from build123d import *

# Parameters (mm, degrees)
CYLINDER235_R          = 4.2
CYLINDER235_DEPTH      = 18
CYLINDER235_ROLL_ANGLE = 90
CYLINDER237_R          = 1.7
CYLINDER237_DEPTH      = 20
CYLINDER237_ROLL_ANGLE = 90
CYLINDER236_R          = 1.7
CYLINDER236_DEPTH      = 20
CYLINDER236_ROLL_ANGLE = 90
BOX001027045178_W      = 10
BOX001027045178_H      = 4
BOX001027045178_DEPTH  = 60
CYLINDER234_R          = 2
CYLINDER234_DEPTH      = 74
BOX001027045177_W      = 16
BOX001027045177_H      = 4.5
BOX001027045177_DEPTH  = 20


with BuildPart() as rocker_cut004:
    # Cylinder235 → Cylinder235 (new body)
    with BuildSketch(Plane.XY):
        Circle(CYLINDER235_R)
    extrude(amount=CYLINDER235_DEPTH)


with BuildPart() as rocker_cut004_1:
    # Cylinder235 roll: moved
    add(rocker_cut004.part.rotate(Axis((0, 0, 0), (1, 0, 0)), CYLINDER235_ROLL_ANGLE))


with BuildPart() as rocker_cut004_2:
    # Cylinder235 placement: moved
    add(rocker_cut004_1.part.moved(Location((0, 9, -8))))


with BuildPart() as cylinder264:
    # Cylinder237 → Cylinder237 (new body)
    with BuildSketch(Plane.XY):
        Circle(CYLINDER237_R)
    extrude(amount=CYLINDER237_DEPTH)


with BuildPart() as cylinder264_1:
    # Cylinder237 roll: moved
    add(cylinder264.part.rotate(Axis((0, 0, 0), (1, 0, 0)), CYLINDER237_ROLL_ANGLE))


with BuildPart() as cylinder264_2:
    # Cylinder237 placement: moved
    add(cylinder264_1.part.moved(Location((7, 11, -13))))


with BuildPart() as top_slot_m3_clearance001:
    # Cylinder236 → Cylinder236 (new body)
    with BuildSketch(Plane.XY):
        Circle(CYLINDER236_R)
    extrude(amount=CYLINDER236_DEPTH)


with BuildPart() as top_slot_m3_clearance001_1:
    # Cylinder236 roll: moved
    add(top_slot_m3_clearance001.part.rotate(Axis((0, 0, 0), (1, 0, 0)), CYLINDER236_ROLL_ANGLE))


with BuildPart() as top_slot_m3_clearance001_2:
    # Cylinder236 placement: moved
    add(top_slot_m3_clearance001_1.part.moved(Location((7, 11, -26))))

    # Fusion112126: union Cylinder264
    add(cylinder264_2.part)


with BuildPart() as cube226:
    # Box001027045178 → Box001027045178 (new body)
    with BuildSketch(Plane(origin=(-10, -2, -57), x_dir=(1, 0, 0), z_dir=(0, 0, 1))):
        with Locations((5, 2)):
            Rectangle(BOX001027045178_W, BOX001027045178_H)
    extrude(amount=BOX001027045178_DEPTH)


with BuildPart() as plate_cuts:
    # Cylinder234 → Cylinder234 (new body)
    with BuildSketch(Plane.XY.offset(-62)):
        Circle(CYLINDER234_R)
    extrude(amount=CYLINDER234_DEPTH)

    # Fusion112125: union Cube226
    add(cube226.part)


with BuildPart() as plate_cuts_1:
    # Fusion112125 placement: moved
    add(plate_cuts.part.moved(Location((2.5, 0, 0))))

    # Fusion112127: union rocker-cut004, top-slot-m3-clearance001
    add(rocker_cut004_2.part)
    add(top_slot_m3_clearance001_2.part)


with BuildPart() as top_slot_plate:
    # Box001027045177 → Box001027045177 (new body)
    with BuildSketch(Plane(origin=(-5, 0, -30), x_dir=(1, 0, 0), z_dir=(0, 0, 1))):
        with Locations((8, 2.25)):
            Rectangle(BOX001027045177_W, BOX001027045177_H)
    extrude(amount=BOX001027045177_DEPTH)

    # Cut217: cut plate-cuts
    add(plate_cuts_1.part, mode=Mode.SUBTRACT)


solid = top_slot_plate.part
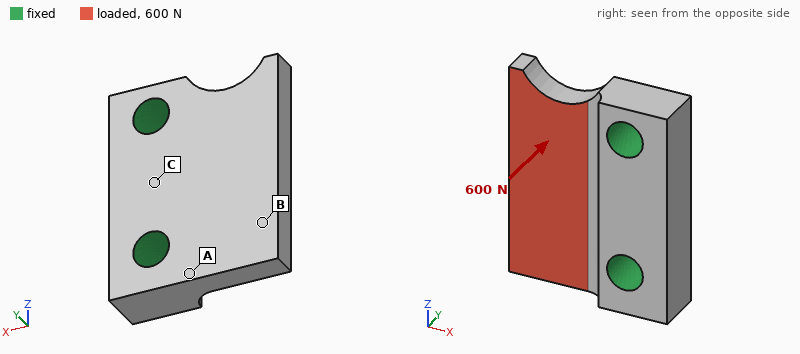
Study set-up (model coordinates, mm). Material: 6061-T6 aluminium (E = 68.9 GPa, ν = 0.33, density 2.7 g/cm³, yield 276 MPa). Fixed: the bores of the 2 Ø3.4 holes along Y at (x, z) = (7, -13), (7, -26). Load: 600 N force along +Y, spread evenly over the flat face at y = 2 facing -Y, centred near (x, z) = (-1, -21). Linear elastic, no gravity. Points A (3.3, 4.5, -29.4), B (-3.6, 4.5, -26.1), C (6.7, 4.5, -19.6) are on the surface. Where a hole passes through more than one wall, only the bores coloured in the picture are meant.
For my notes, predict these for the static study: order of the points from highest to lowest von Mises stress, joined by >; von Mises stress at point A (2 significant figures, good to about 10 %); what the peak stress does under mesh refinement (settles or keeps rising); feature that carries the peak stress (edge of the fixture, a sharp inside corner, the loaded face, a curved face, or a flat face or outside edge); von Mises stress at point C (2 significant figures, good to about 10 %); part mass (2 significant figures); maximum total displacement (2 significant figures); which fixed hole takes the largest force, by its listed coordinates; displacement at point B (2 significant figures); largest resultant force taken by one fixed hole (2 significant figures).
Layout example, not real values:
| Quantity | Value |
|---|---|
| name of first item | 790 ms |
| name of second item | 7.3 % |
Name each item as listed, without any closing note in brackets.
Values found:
| Quantity | Value |
|---|---|
| order of the points from highest to lowest von Mises stress, joined by > | A > C > B |
| von Mises stress at point A | 110 MPa |
| what the peak stress does under mesh refinement | keeps rising |
| feature that carries the peak stress | edge of the fixture |
| von Mises stress at point C | 33 MPa |
| part mass | 2.6 g |
| maximum total displacement | 60 µm |
| which fixed hole takes the largest force, by its listed coordinates | (7, -26) |
| displacement at point B | 47 µm |
| largest resultant force taken by one fixed hole | 340 N |
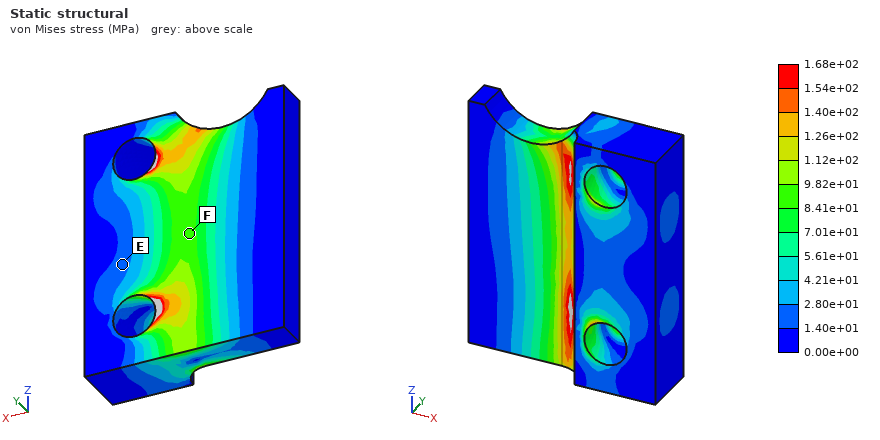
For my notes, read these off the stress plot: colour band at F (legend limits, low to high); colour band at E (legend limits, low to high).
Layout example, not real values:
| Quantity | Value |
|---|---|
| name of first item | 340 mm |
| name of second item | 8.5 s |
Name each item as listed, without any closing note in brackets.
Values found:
| Quantity | Value |
|---|---|
| colour band at F | 8.41e+01 to 9.82e+01 MPa |
| colour band at E | 1.40e+01 to 2.80e+01 MPa |
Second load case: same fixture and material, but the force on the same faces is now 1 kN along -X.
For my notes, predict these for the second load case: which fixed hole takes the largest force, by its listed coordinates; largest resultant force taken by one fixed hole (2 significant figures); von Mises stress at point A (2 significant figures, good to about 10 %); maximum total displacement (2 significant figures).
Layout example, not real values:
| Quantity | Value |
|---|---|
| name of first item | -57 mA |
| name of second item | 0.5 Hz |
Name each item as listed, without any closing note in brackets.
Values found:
| Quantity | Value |
|---|---|
| which fixed hole takes the largest force, by its listed coordinates | (7, -26) |
| largest resultant force taken by one fixed hole | 580 N |
| von Mises stress at point A | 30 MPa |
| maximum total displacement | 26 µm |
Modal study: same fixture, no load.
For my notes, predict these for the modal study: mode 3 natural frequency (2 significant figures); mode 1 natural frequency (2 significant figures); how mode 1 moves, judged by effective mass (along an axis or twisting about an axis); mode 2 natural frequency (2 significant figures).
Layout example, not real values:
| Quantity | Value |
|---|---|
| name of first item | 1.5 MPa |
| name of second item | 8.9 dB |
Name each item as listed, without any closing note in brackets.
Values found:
| Quantity | Value |
|---|---|
| mode 3 natural frequency | 52 kHz |
| mode 1 natural frequency | 20 kHz |
| how mode 1 moves, judged by effective mass | along Y |
| mode 2 natural frequency | 29 kHz |
